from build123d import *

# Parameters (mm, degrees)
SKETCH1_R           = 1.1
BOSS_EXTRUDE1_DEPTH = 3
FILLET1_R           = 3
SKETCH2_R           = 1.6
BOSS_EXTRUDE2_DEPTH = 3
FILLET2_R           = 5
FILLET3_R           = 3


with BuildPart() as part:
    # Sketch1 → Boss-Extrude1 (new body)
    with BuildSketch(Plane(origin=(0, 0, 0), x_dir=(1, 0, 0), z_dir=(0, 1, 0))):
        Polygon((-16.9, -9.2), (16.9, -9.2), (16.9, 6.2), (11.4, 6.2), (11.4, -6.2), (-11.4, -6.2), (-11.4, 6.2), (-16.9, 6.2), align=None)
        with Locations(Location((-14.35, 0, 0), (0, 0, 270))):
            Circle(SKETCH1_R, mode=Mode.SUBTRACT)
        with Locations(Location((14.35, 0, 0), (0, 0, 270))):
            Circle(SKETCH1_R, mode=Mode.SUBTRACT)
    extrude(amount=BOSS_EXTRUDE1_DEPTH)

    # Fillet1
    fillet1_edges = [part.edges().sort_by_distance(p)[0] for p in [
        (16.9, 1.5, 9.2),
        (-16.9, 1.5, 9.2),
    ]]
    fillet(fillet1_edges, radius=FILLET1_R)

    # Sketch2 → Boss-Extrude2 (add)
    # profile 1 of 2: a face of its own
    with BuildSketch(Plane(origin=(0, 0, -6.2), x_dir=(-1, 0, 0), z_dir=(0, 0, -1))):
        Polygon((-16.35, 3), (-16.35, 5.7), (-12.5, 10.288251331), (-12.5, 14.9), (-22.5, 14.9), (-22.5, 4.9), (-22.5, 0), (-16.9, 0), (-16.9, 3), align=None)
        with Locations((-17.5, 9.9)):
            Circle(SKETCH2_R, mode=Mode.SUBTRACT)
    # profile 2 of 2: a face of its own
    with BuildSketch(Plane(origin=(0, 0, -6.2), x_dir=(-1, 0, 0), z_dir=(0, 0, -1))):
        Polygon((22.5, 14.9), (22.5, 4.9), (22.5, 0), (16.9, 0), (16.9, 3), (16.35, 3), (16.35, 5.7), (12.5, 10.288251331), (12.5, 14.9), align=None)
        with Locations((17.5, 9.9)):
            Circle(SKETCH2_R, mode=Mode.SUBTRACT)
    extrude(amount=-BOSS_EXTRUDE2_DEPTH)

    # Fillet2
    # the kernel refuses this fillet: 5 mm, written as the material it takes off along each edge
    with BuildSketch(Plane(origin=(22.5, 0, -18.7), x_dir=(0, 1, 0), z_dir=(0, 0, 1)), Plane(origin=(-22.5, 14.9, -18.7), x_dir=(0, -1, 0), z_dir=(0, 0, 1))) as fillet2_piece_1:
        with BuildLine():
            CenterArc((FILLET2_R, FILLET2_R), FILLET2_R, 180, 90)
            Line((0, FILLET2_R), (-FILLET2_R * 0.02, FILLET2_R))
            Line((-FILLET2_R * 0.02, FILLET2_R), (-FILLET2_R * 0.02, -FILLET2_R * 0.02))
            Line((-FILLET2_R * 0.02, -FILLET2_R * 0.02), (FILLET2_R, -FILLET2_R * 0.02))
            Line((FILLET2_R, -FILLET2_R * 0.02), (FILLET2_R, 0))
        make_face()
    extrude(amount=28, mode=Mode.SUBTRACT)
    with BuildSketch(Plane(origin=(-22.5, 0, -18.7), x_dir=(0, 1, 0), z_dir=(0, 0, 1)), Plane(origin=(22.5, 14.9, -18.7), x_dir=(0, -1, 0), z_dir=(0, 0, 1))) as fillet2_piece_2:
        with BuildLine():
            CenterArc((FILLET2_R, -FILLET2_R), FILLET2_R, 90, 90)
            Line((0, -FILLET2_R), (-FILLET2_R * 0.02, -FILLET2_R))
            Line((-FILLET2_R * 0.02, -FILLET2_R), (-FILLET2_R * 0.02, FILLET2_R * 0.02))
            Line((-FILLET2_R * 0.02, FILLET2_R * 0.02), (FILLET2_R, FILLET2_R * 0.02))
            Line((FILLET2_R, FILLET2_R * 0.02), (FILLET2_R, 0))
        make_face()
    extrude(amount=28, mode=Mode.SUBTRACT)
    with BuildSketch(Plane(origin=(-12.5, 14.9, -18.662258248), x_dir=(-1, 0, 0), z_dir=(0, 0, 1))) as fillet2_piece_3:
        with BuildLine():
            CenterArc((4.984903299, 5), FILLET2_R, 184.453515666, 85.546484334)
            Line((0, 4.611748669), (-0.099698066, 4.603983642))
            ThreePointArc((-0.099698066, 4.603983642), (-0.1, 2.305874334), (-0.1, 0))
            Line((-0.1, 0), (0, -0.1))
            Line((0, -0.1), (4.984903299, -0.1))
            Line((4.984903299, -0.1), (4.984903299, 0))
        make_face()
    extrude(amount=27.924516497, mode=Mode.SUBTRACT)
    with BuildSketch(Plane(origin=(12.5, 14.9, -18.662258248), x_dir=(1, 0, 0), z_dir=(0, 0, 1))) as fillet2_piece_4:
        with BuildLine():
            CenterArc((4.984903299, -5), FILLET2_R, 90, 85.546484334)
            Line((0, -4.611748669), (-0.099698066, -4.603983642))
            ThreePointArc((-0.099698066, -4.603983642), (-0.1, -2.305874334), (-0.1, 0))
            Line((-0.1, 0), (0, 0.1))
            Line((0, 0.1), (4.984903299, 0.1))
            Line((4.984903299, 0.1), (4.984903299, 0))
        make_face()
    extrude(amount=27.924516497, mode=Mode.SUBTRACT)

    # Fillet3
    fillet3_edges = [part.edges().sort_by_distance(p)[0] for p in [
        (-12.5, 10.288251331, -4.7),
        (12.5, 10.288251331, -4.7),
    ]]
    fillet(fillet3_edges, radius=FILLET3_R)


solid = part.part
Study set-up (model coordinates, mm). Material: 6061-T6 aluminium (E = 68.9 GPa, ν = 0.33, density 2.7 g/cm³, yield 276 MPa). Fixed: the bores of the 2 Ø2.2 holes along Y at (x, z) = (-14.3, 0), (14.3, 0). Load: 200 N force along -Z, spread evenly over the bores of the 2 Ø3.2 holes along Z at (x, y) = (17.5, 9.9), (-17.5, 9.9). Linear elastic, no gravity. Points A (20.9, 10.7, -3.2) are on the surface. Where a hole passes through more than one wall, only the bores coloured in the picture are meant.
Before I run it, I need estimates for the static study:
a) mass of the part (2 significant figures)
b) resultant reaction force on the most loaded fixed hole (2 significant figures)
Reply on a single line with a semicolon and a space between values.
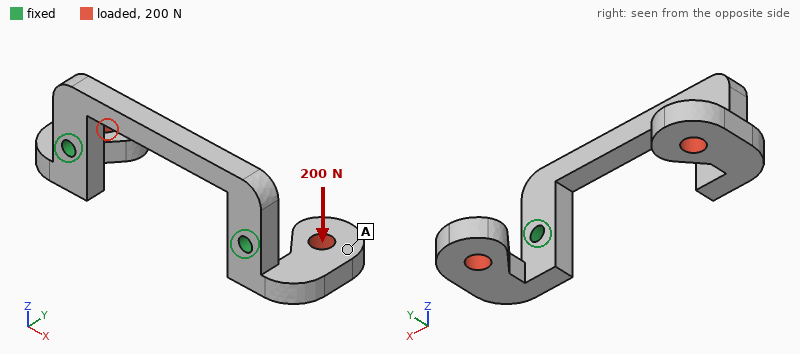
3.3 g; 100 N
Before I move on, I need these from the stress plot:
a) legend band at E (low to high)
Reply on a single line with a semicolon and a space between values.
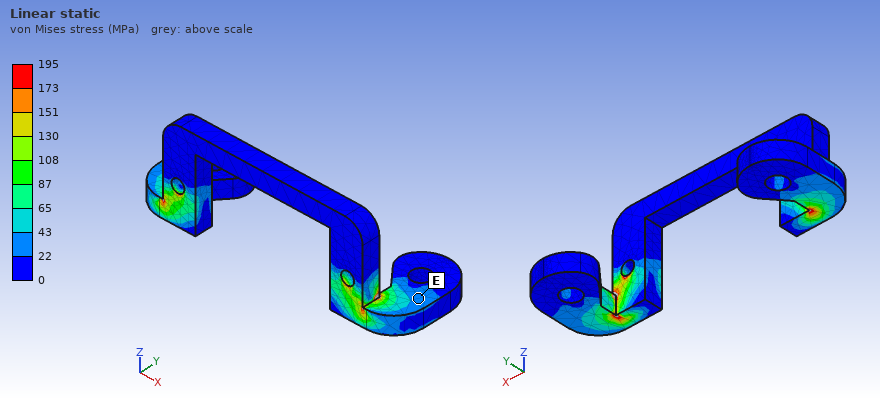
22 to 43 MPa
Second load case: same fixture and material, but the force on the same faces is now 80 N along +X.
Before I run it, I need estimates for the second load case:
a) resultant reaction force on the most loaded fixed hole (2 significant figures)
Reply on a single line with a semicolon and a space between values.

40 N
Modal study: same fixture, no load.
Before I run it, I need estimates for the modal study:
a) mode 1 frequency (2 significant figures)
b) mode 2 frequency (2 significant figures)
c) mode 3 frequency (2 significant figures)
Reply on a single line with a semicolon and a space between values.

6600 Hz; 6600 Hz; 6800 Hz
